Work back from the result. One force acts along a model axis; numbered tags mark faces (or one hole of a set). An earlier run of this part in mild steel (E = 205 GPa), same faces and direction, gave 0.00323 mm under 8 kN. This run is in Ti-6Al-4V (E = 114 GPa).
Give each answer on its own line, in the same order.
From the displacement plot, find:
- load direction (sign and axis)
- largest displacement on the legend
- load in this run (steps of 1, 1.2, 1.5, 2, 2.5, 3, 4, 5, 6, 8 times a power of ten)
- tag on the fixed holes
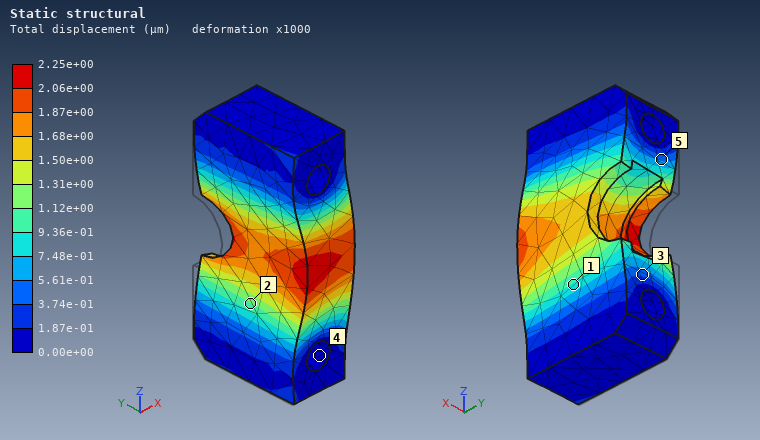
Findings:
+X
2.25e+00 µm
3 kN
4
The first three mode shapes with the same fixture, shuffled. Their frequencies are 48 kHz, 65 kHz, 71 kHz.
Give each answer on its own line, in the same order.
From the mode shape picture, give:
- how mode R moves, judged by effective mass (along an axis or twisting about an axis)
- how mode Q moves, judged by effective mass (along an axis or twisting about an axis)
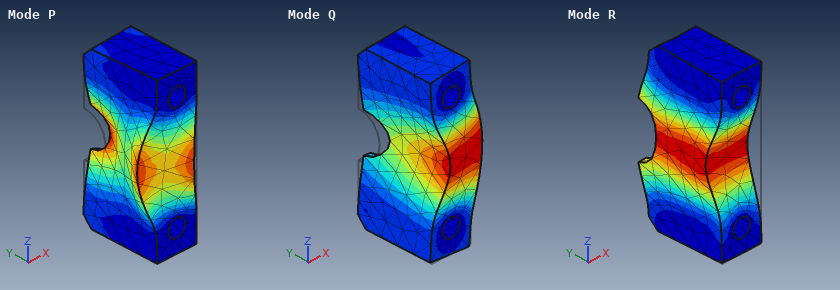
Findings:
along Y
along X
